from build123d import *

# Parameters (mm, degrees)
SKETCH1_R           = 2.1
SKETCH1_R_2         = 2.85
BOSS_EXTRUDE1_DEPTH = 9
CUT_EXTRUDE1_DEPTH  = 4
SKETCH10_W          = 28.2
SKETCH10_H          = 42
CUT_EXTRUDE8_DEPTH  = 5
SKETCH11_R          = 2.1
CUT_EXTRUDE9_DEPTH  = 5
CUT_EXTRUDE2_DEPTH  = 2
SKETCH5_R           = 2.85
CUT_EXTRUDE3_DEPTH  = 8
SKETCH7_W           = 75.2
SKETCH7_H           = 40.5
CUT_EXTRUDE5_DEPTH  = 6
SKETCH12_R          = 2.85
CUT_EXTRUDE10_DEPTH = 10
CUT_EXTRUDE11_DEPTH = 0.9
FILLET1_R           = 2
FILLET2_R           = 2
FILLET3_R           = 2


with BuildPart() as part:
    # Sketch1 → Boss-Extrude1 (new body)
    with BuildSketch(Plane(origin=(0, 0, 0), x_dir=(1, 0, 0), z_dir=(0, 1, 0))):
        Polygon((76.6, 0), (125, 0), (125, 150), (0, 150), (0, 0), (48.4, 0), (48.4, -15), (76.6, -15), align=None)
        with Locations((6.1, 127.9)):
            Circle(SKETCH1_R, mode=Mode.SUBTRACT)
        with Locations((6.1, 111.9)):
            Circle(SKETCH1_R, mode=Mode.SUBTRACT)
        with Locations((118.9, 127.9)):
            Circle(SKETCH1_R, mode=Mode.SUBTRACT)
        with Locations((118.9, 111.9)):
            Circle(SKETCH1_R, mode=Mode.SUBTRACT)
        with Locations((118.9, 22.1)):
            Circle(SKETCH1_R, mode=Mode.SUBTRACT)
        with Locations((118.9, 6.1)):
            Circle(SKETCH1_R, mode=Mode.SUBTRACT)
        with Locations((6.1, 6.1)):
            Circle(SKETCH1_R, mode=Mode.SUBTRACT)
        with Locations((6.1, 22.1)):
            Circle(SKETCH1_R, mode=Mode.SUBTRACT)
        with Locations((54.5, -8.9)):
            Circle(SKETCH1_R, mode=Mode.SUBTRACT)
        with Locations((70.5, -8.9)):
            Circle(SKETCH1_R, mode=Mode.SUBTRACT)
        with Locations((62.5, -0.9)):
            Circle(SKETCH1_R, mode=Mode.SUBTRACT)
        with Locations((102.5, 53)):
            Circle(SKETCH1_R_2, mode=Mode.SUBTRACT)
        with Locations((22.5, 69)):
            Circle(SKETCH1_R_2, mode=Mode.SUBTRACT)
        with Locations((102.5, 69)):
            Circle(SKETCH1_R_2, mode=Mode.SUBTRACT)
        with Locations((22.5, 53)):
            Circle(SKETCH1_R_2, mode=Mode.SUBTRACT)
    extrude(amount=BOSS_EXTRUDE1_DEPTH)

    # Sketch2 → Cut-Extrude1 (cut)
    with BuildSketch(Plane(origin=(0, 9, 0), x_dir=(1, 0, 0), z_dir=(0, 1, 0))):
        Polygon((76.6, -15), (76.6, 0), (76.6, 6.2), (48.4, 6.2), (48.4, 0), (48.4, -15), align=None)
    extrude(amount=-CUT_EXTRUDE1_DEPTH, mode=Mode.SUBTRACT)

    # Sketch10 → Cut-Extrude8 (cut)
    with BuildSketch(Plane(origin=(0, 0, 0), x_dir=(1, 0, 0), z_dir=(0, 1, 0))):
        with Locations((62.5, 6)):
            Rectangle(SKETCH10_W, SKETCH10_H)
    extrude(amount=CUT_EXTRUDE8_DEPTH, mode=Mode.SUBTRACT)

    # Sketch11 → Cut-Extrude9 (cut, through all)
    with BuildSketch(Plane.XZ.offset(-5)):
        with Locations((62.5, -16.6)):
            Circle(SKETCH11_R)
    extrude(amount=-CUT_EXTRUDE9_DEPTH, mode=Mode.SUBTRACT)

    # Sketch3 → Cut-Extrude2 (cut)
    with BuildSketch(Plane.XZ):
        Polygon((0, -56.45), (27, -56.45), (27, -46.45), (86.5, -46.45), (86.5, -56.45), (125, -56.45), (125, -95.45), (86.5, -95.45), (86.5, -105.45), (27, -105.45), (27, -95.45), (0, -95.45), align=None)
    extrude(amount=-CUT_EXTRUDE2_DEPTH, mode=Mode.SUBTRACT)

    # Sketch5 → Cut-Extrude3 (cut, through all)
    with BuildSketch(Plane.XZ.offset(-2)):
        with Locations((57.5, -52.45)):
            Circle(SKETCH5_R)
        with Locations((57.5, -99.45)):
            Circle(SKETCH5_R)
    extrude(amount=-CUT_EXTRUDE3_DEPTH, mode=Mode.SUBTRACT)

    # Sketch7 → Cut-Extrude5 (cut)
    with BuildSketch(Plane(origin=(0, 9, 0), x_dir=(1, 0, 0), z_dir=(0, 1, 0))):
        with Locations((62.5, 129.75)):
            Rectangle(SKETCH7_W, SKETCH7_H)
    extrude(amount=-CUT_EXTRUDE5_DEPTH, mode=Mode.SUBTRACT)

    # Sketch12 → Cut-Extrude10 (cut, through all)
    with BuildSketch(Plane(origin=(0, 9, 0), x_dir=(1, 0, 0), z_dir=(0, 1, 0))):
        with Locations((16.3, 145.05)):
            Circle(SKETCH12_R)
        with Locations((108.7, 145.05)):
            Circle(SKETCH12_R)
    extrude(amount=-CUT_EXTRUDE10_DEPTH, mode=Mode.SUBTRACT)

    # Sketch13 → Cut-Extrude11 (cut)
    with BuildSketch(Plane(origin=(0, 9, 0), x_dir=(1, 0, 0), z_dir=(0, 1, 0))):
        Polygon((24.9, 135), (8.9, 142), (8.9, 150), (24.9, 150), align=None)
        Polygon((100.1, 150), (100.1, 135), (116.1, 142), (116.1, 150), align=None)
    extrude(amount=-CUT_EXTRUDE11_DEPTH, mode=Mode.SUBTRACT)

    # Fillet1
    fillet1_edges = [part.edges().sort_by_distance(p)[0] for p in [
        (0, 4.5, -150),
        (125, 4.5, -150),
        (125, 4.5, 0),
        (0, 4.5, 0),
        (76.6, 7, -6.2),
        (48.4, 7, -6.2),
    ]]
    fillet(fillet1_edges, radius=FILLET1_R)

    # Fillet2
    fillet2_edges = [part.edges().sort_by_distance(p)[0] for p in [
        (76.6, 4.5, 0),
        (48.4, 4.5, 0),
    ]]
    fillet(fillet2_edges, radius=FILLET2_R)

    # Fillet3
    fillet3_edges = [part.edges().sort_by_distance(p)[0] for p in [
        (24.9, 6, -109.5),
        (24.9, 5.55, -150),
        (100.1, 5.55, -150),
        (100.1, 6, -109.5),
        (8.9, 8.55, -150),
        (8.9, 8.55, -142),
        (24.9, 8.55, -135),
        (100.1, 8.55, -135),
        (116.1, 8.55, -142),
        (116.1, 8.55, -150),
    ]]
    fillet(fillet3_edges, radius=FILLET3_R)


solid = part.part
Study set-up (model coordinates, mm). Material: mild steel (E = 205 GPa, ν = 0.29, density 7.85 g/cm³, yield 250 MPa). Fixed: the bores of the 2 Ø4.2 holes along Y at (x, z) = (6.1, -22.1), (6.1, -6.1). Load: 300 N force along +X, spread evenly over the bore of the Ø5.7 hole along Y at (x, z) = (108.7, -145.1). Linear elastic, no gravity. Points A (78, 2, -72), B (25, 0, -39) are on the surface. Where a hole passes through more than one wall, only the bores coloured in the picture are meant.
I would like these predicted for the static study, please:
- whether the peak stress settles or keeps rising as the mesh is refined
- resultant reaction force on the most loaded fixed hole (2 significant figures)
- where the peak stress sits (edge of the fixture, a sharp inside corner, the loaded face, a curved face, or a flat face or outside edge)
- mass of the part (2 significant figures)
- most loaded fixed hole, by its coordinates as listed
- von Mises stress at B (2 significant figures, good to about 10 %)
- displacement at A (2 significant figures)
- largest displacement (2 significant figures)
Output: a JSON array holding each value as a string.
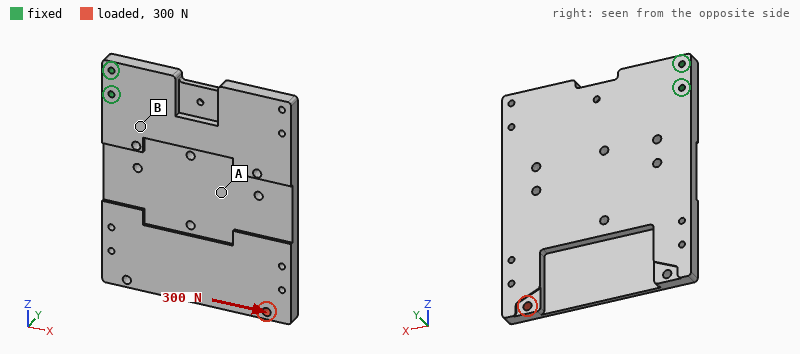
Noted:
["keeps rising", "2.2 kN", "edge of the fixture", "1.0 kg", "(6.1, -22.1)", "4.7 MPa", "17 µm", "37 µm"]
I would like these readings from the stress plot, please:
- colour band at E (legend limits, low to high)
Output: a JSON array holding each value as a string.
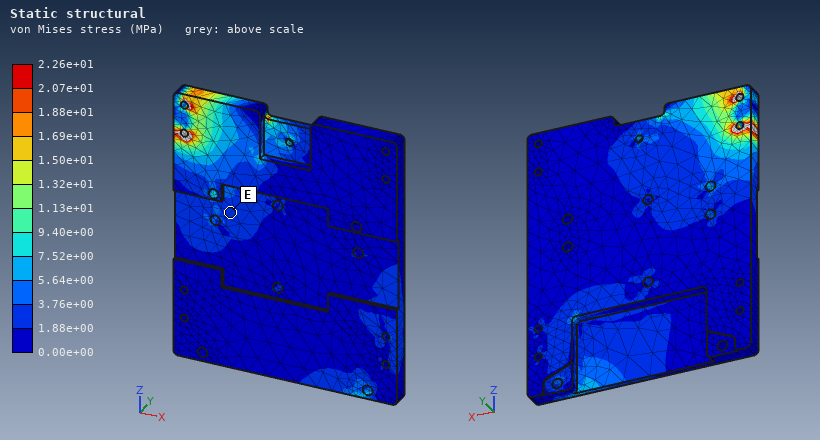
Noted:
["1.88e+00 to 3.76e+00 MPa"]
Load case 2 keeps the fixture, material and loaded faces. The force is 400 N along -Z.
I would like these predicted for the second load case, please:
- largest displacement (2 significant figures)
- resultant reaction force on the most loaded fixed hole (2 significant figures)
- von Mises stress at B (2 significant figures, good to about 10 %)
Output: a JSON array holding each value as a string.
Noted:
["39 µm", "2.2 kN", "4.0 MPa"]
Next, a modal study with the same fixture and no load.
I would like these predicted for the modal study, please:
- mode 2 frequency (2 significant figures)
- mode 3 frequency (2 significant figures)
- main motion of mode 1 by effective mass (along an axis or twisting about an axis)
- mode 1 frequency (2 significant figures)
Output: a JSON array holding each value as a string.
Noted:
["450 Hz", "740 Hz", "along Y", "240 Hz"]
